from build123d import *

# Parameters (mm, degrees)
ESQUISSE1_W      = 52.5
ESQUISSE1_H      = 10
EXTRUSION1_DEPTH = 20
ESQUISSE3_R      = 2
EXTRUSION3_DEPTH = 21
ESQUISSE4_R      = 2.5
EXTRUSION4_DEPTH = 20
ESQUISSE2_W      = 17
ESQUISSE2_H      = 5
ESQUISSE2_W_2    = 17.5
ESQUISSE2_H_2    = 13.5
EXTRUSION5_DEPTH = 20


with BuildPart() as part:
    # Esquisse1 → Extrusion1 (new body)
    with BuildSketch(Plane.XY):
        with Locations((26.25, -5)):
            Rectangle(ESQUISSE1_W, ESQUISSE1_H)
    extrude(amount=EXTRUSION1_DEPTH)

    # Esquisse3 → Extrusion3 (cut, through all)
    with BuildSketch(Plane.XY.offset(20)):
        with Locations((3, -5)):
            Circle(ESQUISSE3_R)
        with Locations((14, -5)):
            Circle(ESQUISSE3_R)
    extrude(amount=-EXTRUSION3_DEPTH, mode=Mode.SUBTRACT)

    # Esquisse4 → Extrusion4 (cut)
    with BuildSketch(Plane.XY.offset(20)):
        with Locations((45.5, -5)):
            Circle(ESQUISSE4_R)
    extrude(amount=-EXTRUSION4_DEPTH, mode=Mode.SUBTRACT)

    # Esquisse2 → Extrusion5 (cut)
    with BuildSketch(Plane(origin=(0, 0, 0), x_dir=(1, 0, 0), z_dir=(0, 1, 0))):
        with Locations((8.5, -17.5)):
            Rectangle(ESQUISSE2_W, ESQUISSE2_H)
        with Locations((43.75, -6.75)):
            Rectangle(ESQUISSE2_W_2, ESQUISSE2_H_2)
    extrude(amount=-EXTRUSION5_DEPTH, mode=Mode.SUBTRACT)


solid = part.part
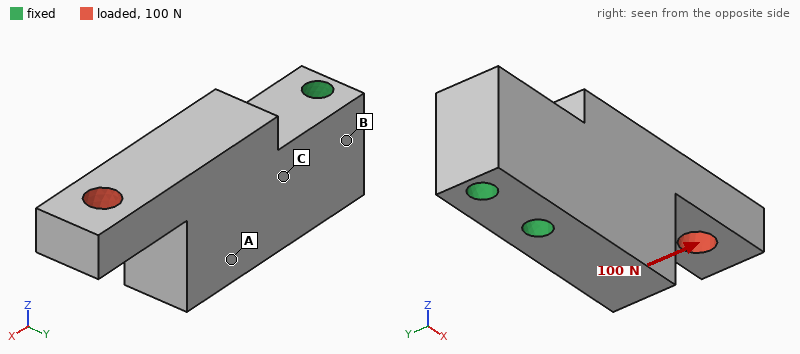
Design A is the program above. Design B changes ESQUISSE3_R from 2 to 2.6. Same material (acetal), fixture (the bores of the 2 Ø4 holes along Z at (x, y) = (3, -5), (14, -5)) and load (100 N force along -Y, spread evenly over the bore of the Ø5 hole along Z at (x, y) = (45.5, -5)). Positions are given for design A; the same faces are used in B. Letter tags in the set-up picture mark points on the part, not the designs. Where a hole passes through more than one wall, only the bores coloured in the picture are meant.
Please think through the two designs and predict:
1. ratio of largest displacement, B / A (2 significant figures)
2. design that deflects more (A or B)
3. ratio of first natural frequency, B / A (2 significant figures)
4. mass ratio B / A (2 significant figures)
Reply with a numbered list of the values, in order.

1. 0.92
2. A
3. 1.1
4. 0.96
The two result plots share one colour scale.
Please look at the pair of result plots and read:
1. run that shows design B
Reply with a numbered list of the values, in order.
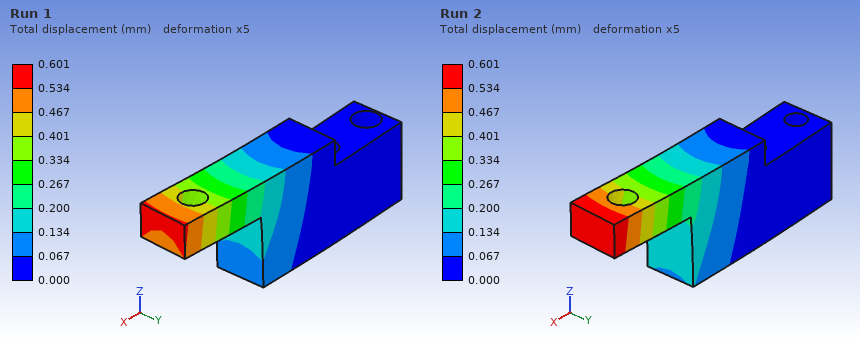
1. Run 1
